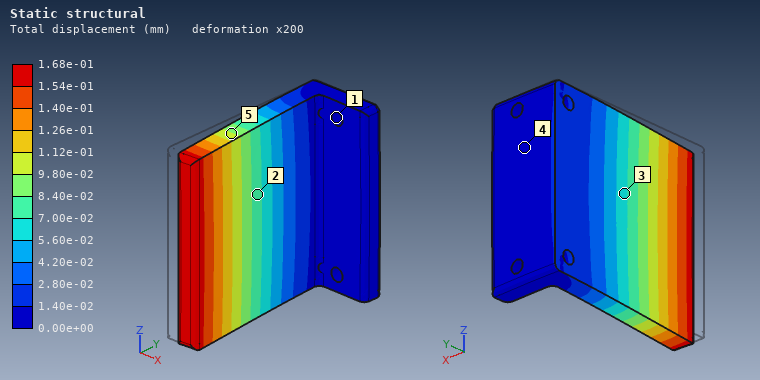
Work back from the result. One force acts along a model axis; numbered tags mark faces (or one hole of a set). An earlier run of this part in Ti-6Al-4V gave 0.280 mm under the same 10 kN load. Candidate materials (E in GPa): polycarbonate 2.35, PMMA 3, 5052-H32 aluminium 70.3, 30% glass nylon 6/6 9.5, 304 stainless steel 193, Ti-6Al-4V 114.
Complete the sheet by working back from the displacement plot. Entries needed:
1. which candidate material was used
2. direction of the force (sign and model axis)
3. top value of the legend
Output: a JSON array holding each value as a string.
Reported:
["304 stainless steel", "+X", "1.68e-01 mm"]
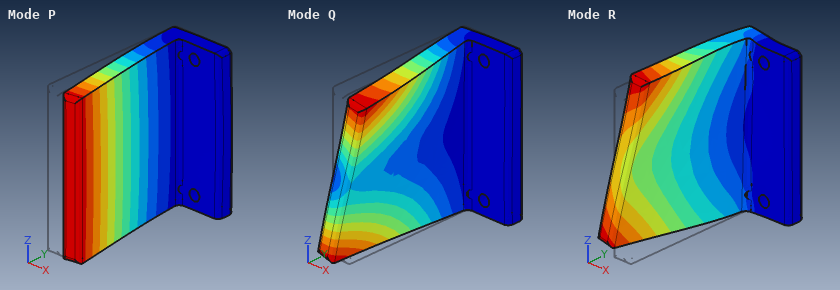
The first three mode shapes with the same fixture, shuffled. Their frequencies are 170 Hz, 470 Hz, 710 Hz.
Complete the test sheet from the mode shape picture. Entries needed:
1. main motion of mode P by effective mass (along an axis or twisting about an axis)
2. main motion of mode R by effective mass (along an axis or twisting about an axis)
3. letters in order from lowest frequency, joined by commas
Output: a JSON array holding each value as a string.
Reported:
["along X", "along Z", "P, Q, R"]
